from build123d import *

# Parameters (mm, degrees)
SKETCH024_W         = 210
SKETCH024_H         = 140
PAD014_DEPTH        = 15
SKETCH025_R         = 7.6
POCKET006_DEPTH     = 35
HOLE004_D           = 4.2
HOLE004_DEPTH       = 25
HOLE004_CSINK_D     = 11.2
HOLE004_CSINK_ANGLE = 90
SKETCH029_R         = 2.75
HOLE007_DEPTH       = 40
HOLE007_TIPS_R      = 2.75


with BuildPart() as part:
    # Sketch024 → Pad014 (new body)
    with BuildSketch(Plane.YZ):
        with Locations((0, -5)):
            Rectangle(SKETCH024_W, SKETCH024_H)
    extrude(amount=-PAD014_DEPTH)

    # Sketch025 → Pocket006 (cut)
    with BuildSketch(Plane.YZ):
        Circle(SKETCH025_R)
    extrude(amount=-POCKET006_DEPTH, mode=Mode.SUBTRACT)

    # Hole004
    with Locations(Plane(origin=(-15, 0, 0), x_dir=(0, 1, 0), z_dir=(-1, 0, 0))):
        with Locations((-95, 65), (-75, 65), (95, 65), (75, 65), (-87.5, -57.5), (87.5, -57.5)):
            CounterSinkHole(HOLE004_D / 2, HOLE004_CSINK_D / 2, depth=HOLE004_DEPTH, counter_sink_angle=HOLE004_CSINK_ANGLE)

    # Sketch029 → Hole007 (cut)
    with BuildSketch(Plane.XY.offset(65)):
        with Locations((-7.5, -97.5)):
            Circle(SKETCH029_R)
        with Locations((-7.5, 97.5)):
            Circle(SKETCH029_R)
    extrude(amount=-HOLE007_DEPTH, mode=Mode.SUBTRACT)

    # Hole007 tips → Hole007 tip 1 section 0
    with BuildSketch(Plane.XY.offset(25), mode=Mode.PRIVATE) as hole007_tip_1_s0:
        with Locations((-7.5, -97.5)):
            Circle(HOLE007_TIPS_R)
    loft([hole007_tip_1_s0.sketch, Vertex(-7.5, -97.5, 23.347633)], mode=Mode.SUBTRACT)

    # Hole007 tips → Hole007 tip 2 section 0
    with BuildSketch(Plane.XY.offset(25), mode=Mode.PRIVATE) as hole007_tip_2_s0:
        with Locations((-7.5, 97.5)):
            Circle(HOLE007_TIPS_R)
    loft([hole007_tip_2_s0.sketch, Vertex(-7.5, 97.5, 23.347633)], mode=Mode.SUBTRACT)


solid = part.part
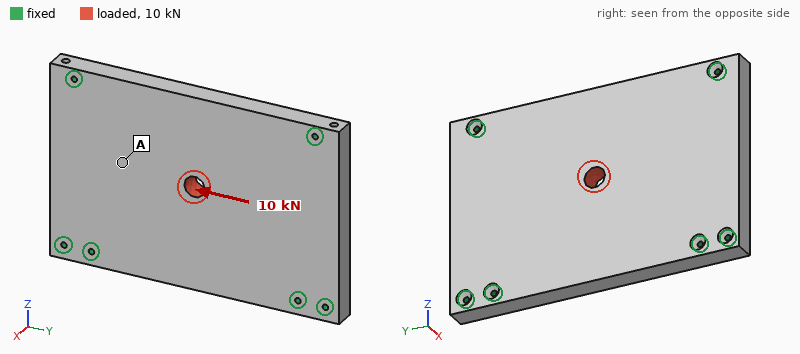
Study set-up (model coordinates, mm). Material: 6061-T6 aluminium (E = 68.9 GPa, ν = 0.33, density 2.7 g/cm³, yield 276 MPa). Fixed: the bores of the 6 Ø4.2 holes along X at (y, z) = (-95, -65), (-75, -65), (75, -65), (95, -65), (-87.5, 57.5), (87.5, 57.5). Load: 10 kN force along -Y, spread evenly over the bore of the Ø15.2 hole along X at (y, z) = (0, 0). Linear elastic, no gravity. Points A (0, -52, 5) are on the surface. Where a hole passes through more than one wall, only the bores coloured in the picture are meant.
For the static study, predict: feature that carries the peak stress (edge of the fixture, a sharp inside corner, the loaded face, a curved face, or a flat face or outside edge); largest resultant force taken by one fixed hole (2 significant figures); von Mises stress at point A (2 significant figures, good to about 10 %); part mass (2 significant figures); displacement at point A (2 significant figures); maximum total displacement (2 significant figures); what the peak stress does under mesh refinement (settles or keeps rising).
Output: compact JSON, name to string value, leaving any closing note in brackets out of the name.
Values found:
{"feature that carries the peak stress": "edge of the fixture", "largest resultant force taken by one fixed hole": "2.4 kN", "von Mises stress at point A": "2.6 MPa", "part mass": "1.2 kg", "displacement at point A": "5.5 µm", "maximum total displacement": "9.9 µm", "what the peak stress does under mesh refinement": "keeps rising"}
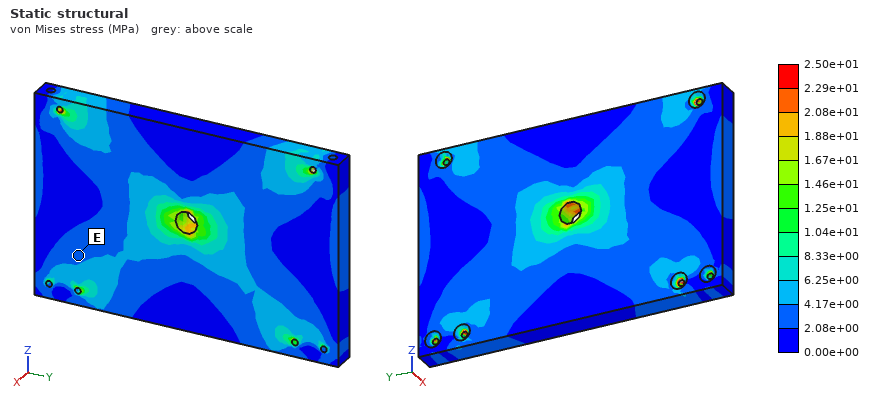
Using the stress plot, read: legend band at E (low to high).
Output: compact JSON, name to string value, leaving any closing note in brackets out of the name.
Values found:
{"legend band at E": "2.08e+00 to 4.17e+00 MPa"}
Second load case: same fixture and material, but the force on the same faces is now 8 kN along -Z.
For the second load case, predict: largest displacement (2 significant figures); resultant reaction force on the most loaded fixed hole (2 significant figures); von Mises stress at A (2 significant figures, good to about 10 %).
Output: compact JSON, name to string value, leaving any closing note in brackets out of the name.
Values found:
{"largest displacement": "11 µm", "resultant reaction force on the most loaded fixed hole": "2.0 kN", "von Mises stress at A": "3.5 MPa"}
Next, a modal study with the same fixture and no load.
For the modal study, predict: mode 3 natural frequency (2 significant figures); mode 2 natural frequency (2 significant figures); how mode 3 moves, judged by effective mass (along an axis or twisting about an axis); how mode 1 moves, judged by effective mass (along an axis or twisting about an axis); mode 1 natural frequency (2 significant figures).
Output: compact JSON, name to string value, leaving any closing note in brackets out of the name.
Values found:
{"mode 3 natural frequency": "3800 Hz", "mode 2 natural frequency": "3100 Hz", "how mode 3 moves, judged by effective mass": "twisting about Z", "how mode 1 moves, judged by effective mass": "along X", "mode 1 natural frequency": "1800 Hz"}
